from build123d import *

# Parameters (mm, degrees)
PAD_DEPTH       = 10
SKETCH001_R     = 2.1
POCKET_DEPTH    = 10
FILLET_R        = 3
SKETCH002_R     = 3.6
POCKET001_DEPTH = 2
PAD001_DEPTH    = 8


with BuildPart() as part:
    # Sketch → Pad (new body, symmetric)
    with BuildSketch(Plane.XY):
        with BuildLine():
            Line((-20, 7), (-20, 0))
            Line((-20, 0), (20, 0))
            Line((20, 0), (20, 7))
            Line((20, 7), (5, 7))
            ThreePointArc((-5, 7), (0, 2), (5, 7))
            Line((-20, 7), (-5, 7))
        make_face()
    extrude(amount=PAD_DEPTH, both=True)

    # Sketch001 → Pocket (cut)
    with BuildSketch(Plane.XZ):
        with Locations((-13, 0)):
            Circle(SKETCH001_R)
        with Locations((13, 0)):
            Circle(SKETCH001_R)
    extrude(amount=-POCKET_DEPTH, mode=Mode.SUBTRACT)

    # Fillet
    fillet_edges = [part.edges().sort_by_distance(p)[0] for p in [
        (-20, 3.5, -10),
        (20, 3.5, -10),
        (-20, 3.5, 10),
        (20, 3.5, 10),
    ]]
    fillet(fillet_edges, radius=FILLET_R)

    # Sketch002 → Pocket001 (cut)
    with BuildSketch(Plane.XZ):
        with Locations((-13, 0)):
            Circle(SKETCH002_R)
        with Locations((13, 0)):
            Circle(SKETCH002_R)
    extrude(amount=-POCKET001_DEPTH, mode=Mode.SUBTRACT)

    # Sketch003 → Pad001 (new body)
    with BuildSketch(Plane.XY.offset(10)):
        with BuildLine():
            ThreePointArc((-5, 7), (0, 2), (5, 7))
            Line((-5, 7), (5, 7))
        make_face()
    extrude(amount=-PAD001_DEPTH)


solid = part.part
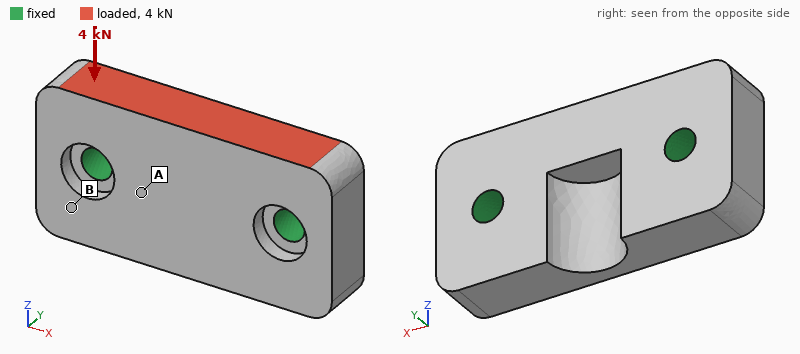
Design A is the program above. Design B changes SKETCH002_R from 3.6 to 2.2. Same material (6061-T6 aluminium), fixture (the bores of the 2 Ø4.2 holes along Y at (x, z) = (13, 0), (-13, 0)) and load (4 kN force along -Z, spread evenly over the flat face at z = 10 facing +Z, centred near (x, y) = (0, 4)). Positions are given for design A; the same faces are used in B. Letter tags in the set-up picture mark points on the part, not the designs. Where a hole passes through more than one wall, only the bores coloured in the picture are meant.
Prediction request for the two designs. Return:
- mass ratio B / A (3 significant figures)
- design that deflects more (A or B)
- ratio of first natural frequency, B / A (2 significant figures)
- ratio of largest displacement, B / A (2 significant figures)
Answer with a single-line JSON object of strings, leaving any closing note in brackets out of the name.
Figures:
{"mass ratio B / A": "1.02", "design that deflects more": "A", "ratio of first natural frequency, B / A": "1.1", "ratio of largest displacement, B / A": "0.86"}
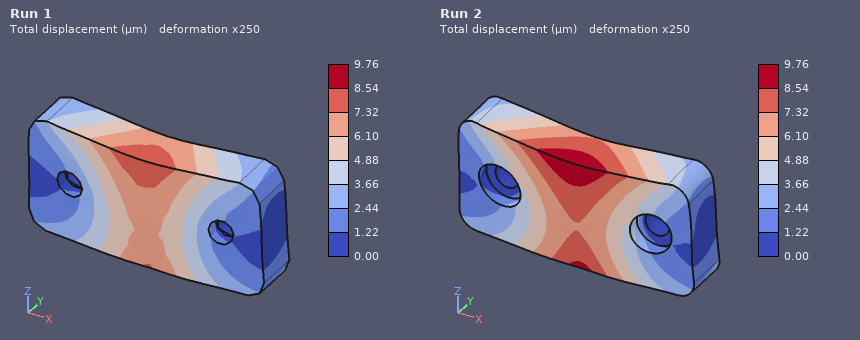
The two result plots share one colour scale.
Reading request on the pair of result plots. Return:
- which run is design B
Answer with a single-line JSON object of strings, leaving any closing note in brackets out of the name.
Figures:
{"which run is design B": "Run 1"}
